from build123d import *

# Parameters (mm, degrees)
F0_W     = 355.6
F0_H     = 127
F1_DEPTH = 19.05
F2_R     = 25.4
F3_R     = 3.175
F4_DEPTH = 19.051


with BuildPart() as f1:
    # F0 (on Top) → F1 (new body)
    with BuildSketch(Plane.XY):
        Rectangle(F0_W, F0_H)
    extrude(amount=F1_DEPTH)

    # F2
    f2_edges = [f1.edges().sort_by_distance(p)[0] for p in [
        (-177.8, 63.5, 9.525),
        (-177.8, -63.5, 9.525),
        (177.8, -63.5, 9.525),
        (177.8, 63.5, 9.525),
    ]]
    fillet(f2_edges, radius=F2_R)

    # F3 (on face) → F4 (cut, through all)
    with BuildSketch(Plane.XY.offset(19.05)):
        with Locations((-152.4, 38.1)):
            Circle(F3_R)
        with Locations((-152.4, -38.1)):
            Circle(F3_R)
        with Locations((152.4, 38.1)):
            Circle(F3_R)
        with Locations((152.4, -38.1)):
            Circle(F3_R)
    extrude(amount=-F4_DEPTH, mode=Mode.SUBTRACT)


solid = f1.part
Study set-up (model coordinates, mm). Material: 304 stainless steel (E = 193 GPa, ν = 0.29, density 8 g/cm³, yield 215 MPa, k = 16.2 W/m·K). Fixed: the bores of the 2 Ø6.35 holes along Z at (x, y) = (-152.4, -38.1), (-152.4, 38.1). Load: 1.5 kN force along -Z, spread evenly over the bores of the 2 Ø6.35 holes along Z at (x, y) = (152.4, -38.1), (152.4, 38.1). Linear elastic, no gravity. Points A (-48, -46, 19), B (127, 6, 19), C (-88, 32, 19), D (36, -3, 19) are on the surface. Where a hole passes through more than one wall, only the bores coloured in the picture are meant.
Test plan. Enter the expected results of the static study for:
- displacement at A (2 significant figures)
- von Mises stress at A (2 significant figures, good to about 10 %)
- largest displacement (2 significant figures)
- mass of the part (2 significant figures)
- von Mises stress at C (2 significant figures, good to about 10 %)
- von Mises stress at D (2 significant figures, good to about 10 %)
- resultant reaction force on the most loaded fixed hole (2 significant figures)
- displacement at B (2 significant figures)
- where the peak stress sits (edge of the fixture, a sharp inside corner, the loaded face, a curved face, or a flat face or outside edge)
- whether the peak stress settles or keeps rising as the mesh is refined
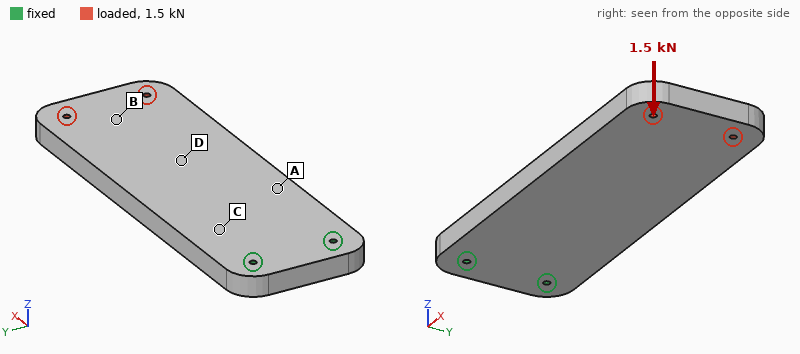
0.20 mm
39 MPa
1.3 mm
6.8 kg
45 MPa
23 MPa
750 N
0.98 mm
edge of the fixture
keeps rising
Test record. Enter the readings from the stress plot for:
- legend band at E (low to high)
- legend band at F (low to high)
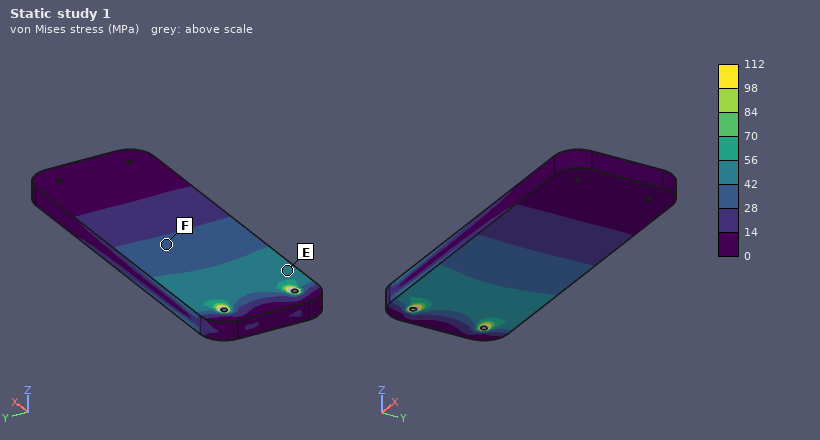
42 to 56 MPa
28 to 42 MPa
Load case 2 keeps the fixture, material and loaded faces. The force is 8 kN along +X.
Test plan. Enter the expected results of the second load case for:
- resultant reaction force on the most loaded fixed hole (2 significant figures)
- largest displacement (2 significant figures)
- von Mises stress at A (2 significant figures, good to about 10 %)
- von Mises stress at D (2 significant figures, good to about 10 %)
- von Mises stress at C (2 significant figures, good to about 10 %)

4.0 kN
6.3 µm
3.3 MPa
3.3 MPa
3.3 MPa
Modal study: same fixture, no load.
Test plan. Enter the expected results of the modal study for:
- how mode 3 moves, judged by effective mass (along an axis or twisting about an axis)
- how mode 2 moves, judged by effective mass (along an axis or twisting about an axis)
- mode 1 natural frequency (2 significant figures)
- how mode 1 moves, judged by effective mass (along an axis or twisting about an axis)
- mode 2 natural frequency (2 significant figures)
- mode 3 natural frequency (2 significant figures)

along Y
twisting about X
130 Hz
along Z
720 Hz
750 Hz
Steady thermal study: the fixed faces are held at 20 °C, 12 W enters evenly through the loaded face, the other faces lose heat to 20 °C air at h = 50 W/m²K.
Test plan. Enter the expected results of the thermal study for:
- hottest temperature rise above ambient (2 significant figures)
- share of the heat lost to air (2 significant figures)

15 K
100 %
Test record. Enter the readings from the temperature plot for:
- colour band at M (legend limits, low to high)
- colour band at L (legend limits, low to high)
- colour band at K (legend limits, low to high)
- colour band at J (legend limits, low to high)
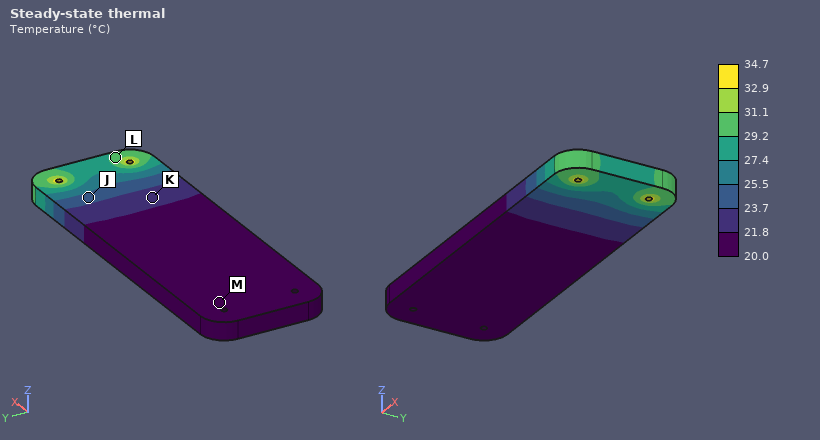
20.0 to 21.8 °C
29.2 to 31.1 °C
21.8 to 23.7 °C
23.7 to 25.5 °C
